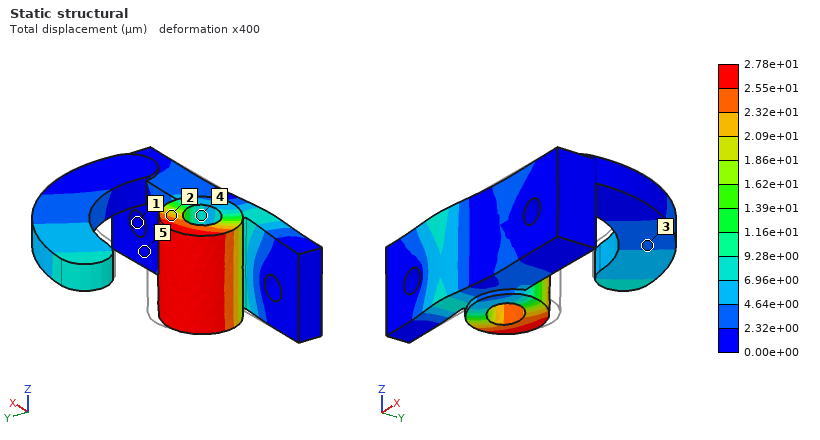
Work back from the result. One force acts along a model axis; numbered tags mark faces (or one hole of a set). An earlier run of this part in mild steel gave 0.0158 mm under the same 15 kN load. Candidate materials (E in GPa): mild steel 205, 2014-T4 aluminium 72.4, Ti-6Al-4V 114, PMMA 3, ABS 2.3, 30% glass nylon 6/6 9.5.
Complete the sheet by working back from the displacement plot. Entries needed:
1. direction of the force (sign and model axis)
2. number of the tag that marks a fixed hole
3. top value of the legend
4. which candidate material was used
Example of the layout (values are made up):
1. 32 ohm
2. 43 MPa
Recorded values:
1. -X
2. 1
3. 2.78e+01 µm
4. Ti-6Al-4V
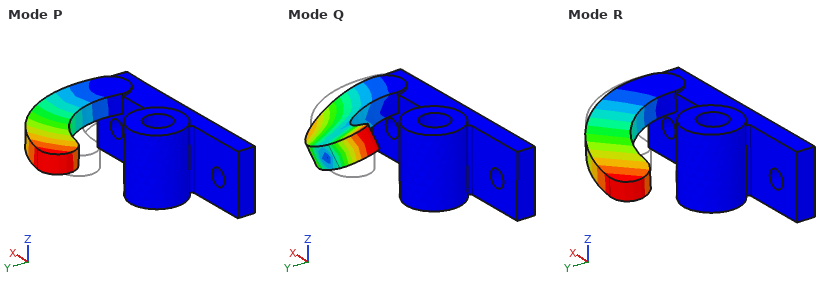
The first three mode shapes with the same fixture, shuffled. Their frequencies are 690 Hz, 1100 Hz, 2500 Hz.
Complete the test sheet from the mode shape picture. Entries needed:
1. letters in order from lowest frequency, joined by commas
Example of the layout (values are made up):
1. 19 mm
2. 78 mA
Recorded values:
1. R, P, Q
